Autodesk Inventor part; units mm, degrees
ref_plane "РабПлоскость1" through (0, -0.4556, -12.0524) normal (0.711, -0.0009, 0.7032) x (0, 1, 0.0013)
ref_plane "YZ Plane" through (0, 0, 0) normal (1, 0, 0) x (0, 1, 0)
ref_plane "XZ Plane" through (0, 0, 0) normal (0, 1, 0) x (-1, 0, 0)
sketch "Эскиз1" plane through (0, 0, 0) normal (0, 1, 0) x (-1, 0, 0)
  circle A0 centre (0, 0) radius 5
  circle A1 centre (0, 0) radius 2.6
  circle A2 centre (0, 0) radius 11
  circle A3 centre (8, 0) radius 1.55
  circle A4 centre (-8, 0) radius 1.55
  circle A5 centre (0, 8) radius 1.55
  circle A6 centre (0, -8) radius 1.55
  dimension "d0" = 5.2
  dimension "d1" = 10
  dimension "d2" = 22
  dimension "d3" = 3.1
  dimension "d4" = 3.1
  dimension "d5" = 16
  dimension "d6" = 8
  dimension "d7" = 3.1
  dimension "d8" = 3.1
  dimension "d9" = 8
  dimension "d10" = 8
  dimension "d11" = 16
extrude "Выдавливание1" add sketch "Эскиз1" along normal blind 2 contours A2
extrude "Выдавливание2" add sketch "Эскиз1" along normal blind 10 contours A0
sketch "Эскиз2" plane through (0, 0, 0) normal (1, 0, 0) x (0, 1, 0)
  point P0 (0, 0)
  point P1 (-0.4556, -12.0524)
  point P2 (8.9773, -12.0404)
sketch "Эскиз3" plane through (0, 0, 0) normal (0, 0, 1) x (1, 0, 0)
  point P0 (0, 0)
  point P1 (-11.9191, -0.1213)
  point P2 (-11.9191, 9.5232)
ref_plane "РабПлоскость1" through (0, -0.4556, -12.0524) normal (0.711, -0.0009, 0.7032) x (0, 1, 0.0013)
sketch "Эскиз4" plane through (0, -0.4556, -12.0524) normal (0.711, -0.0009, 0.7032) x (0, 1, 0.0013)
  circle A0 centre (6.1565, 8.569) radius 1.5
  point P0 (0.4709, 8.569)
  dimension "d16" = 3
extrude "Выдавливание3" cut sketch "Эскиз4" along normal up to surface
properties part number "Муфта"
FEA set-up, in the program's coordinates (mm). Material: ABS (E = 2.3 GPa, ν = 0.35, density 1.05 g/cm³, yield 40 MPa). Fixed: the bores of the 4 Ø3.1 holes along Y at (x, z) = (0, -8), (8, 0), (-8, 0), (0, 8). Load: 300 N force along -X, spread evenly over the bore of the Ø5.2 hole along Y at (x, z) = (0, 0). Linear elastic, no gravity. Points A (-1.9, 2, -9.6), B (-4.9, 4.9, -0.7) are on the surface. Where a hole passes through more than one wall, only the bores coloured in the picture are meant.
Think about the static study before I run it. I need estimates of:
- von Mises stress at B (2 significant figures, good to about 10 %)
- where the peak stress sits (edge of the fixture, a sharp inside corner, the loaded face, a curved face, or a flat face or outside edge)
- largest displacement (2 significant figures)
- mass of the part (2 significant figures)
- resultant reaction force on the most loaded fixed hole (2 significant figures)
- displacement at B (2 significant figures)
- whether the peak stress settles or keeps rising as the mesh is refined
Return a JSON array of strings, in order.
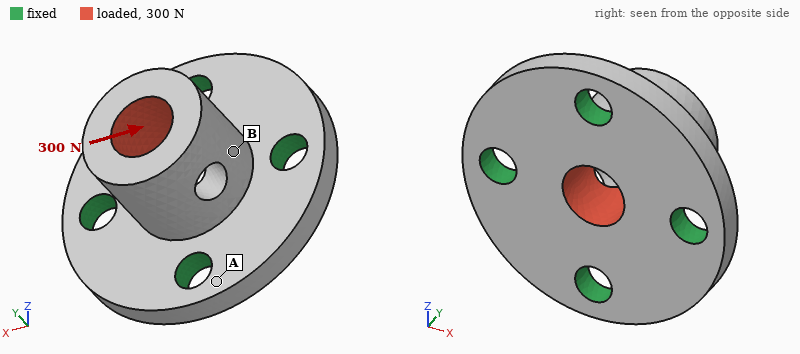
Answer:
["8.4 MPa", "edge of the fixture", "0.13 mm", "1.2 g", "140 N", "0.071 mm", "keeps rising"]
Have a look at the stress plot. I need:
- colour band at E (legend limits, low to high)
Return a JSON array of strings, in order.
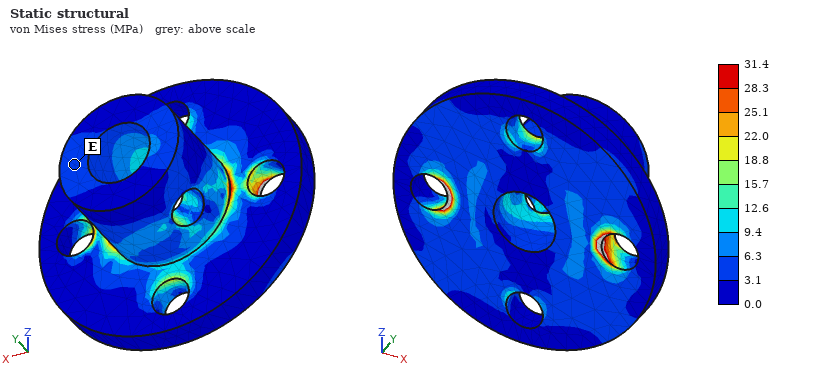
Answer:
["3.1 to 6.3 MPa"]
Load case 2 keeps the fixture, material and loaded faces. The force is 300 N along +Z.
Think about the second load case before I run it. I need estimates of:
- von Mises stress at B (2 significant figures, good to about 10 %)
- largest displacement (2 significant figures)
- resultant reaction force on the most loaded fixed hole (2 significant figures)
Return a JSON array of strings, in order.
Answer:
["7.2 MPa", "0.13 mm", "140 N"]
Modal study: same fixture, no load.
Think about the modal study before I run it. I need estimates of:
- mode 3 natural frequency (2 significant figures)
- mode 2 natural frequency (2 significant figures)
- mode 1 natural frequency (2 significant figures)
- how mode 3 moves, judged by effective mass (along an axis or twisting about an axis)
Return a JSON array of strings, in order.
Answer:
["17 kHz", "12 kHz", "11 kHz", "along Y"]
